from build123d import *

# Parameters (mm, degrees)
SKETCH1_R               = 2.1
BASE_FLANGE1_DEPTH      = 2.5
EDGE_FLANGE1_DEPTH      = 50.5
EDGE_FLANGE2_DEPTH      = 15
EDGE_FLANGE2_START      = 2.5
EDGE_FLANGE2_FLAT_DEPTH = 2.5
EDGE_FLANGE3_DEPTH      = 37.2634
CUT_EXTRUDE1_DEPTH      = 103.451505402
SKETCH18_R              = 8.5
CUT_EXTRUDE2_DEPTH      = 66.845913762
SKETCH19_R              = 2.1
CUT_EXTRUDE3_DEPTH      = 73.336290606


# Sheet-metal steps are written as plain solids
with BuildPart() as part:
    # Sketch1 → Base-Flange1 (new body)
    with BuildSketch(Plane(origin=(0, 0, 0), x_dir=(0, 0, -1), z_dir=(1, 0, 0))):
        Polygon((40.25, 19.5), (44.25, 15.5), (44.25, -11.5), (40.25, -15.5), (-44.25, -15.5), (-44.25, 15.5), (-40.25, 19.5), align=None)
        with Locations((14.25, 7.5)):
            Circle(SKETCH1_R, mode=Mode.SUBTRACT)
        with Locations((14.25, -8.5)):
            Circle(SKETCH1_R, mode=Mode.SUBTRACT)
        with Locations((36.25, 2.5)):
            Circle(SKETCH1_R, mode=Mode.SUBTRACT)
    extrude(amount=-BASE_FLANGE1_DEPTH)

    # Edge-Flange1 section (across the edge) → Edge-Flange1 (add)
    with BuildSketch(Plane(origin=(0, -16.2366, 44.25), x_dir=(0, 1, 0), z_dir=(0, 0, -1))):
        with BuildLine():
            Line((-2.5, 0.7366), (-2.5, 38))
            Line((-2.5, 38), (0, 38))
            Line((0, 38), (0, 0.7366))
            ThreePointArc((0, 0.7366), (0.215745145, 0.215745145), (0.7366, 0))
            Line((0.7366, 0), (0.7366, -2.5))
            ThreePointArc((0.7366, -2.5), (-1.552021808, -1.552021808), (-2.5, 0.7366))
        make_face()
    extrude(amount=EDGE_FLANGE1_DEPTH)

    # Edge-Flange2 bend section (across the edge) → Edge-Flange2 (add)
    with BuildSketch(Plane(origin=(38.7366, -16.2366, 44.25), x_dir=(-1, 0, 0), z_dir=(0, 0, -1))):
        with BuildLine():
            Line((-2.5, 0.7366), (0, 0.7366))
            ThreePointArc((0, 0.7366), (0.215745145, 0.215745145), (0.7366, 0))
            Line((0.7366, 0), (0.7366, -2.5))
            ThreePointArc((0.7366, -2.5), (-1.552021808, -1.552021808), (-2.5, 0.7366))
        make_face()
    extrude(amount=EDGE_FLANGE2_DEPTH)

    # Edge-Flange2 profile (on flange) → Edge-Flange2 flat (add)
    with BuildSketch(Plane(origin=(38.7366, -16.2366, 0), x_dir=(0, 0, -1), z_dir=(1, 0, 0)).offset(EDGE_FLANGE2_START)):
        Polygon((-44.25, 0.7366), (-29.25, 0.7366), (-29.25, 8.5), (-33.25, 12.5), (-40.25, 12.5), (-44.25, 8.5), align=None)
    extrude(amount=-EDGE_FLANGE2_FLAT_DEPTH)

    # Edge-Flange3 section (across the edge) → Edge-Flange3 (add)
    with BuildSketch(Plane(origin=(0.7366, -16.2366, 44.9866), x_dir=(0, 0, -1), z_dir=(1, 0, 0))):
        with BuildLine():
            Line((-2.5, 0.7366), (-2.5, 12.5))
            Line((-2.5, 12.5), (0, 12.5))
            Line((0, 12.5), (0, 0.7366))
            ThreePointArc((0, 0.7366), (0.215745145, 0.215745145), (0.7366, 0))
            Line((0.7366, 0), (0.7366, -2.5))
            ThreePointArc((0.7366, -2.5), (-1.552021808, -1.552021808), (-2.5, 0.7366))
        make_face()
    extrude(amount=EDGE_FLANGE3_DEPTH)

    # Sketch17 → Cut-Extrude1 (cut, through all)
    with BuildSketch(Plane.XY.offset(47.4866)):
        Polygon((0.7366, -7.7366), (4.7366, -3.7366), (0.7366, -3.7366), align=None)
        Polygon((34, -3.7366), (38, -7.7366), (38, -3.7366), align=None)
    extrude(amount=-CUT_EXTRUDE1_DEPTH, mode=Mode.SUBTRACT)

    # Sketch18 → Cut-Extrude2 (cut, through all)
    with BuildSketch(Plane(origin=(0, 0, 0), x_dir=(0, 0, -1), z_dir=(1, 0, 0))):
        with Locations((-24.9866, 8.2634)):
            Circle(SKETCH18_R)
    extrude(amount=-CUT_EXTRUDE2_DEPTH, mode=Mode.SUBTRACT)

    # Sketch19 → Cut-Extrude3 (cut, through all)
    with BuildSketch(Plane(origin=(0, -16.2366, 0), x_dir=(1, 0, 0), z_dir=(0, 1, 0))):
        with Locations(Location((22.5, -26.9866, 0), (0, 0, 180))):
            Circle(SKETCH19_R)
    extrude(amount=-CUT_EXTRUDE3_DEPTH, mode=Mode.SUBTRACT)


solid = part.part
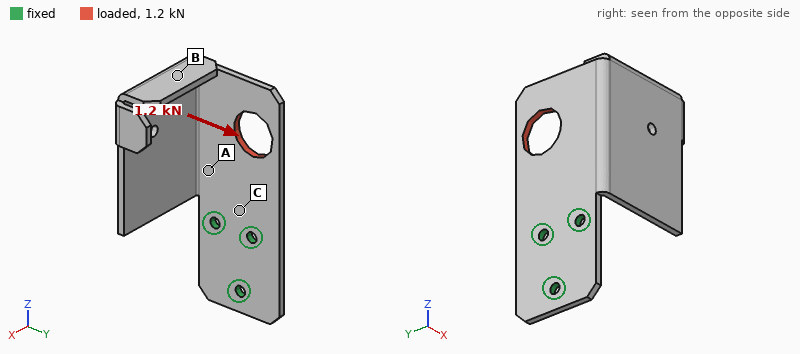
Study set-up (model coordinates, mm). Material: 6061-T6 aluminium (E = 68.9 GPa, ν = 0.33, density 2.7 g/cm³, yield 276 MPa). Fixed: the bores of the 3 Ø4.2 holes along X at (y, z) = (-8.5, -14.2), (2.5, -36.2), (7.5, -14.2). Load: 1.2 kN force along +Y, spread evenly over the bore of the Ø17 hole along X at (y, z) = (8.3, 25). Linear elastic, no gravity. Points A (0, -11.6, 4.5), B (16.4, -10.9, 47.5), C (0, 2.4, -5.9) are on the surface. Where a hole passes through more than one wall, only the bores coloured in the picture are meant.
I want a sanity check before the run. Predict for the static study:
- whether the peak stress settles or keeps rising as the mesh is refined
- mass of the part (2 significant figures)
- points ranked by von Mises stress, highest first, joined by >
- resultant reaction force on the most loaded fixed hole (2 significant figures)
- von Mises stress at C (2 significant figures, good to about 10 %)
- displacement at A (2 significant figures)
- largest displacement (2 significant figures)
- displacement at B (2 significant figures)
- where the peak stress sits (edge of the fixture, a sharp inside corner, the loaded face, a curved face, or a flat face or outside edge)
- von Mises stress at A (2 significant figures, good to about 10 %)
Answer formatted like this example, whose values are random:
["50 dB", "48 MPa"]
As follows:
["keeps rising", "38 g", "C > A > B", "2.1 kN", "52 MPa", "0.035 mm", "0.14 mm", "0.13 mm", "edge of the fixture", "26 MPa"]
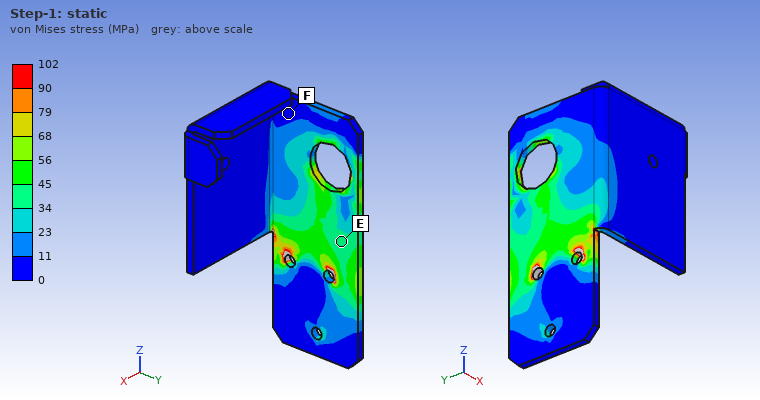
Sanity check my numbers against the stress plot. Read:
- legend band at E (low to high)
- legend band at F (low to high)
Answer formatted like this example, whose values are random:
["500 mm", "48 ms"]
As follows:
["34 to 45 MPa", "0 to 11 MPa"]
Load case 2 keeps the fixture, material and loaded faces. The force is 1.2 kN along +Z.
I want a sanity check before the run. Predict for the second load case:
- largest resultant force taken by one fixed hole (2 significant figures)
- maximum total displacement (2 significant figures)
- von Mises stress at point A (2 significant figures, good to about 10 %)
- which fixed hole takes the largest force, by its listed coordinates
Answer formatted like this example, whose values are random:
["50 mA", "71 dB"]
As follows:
["930 N", "38 µm", "3.8 MPa", "(7.5, -14.2)"]
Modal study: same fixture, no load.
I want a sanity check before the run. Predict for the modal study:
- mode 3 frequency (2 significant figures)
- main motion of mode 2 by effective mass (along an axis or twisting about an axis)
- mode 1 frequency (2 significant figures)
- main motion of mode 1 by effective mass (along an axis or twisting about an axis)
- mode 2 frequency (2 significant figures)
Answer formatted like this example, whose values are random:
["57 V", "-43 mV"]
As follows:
["1700 Hz", "along Y", "310 Hz", "along X", "540 Hz"]
